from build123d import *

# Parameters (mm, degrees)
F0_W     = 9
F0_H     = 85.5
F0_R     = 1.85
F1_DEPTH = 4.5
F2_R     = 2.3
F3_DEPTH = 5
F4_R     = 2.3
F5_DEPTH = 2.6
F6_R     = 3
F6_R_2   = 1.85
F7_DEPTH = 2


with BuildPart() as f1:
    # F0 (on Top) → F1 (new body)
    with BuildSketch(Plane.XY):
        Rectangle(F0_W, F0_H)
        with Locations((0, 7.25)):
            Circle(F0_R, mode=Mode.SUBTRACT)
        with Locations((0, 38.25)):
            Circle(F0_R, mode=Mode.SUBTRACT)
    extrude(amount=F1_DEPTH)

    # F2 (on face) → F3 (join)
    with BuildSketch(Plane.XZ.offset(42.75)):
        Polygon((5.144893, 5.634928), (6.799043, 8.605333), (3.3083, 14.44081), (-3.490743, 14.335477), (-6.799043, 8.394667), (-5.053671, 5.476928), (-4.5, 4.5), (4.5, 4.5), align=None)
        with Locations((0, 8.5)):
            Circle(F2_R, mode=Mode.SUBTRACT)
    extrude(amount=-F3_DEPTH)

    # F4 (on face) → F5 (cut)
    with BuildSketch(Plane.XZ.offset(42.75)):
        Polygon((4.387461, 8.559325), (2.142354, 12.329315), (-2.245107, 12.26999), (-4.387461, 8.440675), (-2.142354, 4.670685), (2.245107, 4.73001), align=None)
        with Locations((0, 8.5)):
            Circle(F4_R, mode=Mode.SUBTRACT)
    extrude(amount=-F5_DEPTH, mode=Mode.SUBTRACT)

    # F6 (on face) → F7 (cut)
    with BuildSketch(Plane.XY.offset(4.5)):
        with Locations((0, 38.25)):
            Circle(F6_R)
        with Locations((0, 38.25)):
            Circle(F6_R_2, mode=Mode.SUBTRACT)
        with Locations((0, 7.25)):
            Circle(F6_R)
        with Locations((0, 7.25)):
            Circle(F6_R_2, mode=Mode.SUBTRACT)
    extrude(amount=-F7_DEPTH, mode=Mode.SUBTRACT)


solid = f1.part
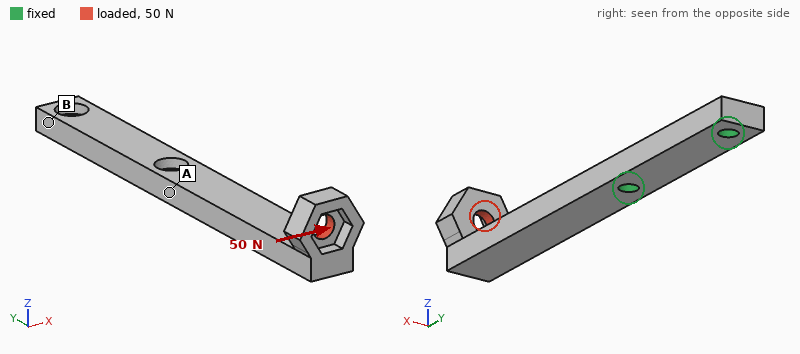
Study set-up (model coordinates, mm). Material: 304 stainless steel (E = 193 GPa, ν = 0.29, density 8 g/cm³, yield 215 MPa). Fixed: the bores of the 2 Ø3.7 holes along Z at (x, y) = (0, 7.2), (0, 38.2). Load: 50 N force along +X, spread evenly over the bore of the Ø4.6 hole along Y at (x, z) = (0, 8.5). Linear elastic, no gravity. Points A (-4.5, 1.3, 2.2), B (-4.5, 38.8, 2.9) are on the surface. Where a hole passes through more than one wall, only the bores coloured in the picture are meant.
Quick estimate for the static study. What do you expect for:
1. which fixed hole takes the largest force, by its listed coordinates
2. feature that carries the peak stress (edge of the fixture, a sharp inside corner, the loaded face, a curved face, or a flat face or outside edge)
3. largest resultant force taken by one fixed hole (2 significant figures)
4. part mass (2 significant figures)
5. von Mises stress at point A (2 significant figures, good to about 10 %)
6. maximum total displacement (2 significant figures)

(0, 7.2)
edge of the fixture
80 N
29 g
35 MPa
56 µm
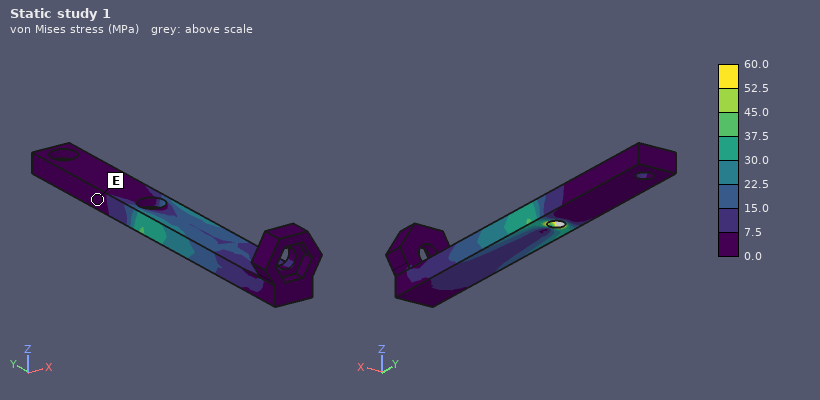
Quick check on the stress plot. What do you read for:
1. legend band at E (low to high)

0.0 to 7.5 MPa
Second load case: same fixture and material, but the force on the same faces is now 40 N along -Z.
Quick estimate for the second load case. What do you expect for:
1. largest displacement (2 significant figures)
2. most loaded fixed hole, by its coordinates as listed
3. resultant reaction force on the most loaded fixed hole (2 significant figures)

0.14 mm
(0, 7.2)
83 N
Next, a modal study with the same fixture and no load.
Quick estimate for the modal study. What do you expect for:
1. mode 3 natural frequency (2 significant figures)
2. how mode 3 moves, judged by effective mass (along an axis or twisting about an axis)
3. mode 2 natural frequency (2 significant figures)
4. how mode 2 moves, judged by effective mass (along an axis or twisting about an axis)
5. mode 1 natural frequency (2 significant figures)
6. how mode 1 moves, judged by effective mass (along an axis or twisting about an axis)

5800 Hz
twisting about Y
2000 Hz
along X
1000 Hz
along Z
